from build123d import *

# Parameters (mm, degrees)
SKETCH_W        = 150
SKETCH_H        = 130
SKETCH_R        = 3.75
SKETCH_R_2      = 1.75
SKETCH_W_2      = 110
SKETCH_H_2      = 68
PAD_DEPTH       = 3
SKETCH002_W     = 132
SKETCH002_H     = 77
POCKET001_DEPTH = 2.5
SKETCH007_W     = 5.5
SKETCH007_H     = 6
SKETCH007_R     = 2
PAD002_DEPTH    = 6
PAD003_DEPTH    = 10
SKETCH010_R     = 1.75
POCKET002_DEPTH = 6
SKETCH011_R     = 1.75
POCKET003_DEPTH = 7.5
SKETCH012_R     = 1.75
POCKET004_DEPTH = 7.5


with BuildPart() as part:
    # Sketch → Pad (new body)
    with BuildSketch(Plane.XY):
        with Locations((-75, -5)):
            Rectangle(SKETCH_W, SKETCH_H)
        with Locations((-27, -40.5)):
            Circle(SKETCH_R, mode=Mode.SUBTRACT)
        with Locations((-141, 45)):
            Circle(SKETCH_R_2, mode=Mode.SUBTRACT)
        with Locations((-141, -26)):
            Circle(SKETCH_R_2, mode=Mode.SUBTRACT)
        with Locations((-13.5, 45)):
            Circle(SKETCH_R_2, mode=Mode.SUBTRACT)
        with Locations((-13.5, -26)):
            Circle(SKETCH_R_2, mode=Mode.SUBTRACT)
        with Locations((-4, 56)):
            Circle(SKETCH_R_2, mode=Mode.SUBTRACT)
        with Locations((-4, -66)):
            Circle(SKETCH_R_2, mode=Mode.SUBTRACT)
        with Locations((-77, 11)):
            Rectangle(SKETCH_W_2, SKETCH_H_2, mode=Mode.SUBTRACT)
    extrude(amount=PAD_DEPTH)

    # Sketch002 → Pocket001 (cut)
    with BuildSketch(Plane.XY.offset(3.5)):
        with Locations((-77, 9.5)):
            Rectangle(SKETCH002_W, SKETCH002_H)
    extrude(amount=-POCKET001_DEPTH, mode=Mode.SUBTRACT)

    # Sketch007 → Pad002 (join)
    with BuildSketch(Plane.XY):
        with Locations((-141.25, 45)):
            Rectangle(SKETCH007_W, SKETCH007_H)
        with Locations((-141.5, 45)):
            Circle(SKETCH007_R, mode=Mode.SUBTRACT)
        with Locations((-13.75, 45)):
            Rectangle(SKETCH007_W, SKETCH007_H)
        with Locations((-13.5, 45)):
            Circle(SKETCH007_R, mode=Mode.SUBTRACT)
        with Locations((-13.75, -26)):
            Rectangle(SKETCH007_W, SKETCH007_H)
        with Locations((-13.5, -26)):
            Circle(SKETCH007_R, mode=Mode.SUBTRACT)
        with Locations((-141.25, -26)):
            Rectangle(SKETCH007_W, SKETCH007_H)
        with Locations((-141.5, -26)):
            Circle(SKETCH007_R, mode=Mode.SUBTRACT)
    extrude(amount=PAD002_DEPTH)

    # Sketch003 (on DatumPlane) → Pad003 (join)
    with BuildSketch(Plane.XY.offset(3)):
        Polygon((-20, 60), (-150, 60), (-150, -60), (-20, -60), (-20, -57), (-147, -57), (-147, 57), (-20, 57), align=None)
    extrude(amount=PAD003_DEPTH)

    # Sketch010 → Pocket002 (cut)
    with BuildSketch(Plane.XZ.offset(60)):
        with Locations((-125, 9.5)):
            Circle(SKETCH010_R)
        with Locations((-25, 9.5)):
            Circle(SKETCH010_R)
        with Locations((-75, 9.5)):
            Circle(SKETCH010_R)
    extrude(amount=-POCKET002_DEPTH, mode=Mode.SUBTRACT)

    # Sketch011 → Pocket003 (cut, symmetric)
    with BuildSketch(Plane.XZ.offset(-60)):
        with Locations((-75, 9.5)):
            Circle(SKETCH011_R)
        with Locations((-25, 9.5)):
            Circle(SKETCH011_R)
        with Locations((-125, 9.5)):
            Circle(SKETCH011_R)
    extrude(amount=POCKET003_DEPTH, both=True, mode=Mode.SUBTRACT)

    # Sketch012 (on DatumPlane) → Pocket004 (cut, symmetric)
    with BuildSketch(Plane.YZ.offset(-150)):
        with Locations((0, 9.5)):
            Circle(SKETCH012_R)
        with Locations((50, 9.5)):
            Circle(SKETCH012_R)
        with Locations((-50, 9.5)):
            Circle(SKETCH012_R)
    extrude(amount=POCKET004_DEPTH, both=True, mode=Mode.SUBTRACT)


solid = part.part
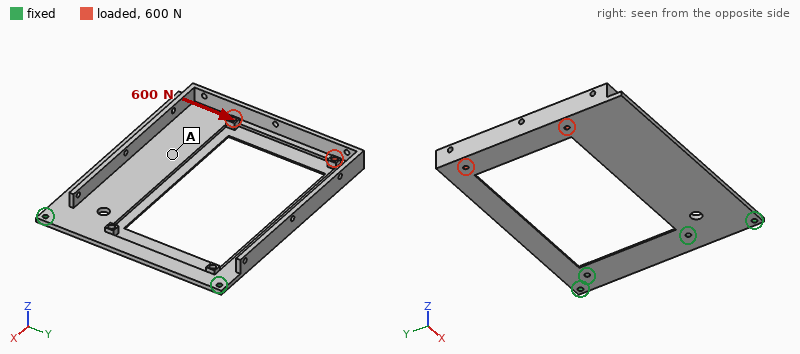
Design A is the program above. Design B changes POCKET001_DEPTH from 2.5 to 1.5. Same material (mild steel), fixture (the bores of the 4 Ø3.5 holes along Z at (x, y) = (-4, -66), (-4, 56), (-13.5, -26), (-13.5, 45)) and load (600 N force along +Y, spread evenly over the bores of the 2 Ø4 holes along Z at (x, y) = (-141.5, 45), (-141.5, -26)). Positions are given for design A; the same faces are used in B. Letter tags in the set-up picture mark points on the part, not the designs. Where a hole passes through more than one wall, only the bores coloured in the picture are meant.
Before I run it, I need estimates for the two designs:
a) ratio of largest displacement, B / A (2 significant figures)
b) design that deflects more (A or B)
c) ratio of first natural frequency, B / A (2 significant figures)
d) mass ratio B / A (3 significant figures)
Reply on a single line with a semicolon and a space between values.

0.80; A; 1.0; 1.06
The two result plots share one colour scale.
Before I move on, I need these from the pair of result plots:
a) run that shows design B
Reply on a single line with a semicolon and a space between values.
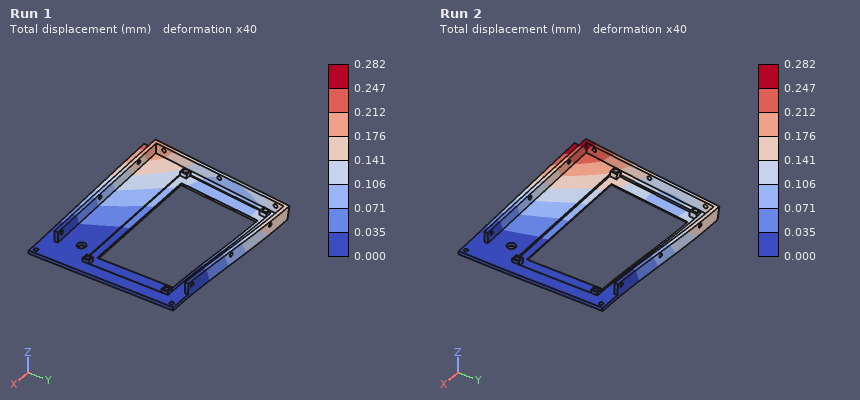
Run 1
